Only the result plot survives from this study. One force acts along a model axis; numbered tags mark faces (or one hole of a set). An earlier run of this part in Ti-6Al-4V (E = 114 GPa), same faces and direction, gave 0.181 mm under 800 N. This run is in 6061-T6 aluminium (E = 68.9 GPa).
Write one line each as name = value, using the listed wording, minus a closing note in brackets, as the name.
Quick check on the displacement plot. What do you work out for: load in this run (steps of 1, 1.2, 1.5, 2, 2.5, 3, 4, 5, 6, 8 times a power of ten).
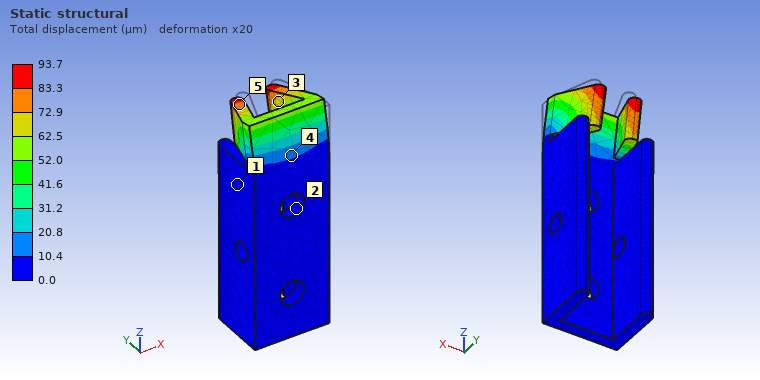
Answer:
load in this run = 250 N
